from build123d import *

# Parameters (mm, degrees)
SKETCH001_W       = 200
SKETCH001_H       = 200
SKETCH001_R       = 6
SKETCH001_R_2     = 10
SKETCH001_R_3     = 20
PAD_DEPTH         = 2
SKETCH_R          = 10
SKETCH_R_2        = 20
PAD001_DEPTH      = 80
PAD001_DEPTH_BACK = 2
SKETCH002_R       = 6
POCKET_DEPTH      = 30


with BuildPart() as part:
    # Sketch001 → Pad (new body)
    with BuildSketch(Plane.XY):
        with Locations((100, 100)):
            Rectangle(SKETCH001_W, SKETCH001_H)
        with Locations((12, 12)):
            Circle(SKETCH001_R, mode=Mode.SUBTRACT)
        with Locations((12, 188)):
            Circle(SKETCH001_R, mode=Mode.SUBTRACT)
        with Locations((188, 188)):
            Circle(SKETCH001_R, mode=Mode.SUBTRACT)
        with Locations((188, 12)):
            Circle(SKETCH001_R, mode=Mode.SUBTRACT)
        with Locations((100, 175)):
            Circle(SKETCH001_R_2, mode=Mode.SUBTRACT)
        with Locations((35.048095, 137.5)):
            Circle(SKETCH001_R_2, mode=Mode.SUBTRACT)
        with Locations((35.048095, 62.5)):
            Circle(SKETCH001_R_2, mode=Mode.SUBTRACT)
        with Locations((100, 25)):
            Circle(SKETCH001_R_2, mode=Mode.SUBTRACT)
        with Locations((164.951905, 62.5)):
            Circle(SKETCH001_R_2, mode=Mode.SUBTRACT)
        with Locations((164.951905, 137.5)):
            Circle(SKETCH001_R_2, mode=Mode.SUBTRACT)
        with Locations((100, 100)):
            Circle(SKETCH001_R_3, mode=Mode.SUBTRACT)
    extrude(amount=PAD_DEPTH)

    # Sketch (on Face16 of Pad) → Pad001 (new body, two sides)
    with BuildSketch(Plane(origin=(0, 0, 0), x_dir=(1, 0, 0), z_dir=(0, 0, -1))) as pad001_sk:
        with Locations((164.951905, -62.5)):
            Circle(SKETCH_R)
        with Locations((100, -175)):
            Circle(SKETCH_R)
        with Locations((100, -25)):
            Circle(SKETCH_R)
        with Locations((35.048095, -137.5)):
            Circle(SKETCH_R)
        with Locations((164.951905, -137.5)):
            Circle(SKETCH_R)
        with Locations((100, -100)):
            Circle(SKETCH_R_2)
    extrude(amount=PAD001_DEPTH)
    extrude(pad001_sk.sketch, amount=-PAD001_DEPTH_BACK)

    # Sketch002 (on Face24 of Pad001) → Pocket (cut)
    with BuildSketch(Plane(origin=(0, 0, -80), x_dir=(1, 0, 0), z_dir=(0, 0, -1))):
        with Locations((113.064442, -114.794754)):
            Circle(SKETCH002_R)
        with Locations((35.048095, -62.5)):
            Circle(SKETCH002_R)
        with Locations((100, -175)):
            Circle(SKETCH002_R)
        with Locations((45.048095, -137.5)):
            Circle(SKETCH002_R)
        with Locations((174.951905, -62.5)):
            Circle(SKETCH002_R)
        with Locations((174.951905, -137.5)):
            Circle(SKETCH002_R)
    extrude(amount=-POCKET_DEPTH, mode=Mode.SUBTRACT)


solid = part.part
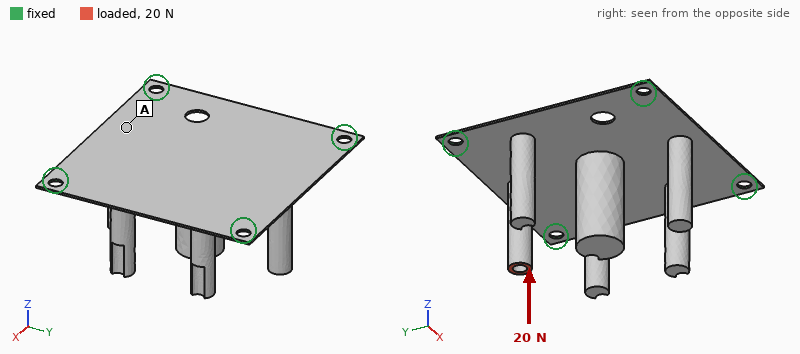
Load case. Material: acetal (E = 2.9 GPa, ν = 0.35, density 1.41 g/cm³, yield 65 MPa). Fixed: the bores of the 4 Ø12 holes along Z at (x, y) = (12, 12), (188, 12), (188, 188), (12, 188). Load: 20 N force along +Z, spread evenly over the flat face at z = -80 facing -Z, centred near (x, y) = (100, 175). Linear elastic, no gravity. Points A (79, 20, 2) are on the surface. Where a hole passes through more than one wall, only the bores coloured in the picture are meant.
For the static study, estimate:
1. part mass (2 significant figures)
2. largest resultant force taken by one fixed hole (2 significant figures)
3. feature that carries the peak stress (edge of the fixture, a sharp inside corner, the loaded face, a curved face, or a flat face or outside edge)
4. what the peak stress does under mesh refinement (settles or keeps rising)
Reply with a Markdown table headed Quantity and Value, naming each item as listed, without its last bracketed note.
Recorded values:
| Quantity | Value |
|---|---|
| part mass | 420 g |
| largest resultant force taken by one fixed hole | 10 N |
| feature that carries the peak stress | edge of the fixture |
| what the peak stress does under mesh refinement | keeps rising |
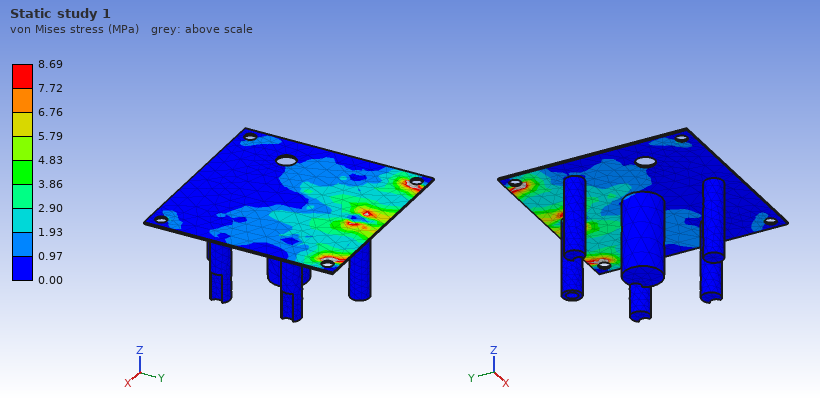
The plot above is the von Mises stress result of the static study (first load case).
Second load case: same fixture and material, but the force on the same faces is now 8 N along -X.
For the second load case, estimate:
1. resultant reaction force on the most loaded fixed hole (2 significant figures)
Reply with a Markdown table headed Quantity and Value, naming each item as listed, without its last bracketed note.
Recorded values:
| Quantity | Value |
|---|---|
| resultant reaction force on the most loaded fixed hole | 5.7 N |
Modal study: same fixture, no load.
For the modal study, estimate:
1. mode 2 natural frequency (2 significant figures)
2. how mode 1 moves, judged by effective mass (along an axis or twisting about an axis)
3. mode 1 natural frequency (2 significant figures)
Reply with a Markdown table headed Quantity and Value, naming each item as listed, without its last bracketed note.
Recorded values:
| Quantity | Value |
|---|---|
| mode 2 natural frequency | 39 Hz |
| how mode 1 moves, judged by effective mass | along Z |
| mode 1 natural frequency | 27 Hz |
